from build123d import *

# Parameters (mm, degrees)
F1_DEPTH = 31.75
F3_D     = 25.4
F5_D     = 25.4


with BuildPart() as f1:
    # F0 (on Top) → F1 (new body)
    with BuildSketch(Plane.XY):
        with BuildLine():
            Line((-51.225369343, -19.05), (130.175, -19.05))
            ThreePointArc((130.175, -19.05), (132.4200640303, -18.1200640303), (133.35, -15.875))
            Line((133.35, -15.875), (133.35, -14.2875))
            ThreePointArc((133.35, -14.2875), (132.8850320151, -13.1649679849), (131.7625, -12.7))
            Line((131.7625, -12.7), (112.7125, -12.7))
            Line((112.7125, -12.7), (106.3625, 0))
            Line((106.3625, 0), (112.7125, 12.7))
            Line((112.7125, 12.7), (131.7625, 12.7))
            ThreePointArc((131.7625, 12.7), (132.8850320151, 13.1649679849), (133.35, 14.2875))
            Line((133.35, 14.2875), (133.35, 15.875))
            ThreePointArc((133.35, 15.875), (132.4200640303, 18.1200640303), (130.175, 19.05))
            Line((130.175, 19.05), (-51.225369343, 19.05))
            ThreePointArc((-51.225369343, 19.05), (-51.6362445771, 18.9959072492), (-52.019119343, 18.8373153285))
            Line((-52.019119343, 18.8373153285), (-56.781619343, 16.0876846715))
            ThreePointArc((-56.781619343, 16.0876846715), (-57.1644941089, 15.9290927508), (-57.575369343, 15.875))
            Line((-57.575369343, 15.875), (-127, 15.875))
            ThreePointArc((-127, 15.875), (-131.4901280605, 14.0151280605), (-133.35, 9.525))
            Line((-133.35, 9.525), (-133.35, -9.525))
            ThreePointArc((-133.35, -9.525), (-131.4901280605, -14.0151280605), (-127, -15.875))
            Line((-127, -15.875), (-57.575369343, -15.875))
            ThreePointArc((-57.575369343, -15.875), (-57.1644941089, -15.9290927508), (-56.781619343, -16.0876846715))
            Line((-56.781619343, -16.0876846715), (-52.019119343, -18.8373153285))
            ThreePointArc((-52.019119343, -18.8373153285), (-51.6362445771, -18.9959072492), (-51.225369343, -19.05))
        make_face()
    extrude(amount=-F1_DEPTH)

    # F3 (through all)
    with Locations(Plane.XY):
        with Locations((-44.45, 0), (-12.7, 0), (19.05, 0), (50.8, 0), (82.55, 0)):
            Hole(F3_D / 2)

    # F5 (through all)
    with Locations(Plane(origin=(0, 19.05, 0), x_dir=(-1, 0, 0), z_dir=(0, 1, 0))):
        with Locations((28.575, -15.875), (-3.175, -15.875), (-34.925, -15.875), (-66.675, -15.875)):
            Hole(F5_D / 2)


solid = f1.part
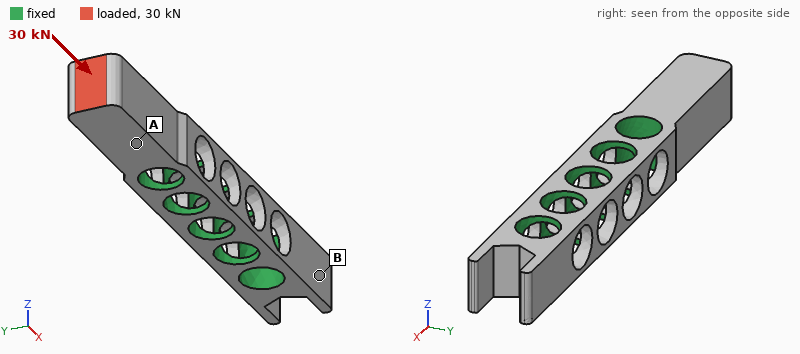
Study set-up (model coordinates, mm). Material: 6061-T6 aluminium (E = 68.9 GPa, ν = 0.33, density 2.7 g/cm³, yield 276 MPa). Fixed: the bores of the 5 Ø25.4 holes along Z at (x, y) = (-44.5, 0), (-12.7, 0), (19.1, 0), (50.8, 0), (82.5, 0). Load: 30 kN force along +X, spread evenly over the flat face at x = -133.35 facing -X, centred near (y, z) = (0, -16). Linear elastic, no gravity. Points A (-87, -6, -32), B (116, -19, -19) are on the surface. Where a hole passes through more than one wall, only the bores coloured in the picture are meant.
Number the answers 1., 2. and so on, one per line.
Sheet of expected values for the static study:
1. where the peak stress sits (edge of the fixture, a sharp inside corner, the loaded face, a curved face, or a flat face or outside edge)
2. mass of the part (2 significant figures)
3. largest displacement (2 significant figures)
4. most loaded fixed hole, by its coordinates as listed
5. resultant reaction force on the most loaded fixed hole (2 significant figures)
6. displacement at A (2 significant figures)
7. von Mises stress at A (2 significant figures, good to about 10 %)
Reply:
1. the loaded face
2. 410 g
3. 39 µm
4. (-44.5, 0)
5. 30 kN
6. 14 µm
7. 30 MPa
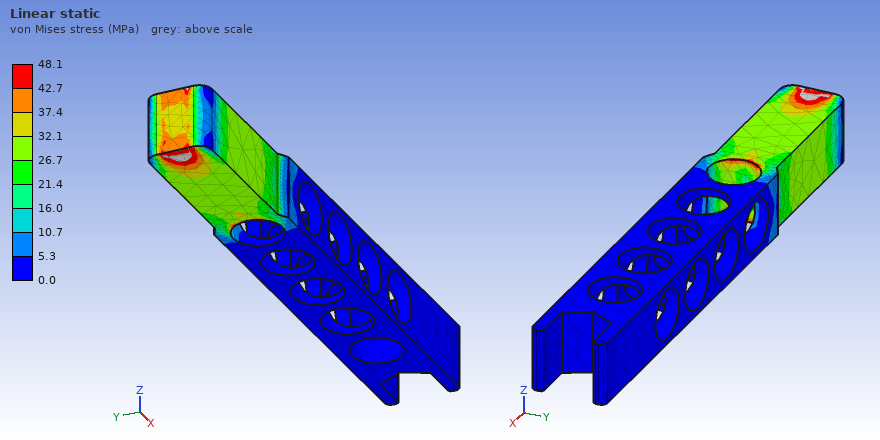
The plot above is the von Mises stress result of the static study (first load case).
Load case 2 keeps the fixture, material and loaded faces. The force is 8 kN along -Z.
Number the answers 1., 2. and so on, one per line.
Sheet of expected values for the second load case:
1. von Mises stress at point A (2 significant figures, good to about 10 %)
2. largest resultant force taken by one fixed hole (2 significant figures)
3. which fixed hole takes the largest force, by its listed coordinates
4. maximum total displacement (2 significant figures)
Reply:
1. 69 MPa
2. 8.0 kN
3. (-44.5, 0)
4. 0.26 mm
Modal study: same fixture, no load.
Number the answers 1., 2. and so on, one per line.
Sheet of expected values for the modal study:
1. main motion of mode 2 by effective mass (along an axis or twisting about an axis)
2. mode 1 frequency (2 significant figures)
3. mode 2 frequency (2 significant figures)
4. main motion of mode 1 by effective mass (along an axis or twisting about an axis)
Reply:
1. along Z
2. 3600 Hz
3. 3800 Hz
4. along Y
